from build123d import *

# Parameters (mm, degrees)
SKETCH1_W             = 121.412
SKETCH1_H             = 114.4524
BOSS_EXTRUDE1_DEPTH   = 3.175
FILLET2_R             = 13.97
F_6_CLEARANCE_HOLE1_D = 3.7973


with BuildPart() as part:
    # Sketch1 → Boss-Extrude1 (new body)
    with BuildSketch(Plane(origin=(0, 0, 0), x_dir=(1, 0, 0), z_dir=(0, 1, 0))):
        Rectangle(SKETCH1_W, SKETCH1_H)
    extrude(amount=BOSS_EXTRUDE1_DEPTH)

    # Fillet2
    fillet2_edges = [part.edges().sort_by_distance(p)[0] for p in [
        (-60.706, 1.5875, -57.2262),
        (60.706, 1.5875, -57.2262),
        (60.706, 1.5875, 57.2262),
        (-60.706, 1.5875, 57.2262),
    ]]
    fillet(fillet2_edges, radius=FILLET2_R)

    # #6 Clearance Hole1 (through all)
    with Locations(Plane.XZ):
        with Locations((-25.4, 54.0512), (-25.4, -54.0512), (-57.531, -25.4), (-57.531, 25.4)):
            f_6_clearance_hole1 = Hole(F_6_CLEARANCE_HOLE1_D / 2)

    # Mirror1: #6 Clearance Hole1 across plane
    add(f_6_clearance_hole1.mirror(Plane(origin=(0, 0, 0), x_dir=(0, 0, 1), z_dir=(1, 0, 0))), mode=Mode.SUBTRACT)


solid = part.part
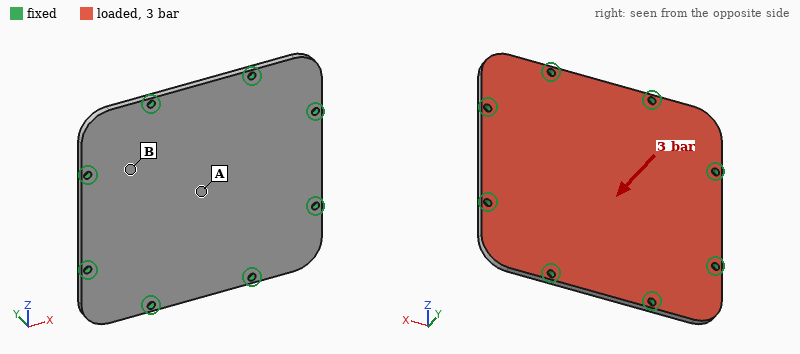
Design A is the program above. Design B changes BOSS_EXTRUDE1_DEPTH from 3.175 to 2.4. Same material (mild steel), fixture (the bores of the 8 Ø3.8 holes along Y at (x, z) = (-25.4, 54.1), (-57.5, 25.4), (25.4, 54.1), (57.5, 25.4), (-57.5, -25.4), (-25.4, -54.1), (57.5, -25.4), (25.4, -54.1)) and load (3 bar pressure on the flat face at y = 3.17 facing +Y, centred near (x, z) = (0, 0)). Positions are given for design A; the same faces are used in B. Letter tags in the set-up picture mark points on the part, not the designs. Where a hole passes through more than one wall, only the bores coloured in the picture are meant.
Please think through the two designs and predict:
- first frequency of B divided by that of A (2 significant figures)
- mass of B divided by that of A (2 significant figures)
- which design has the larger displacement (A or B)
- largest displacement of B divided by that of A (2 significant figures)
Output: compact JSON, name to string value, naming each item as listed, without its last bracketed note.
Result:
{"first frequency of B divided by that of A": "0.77", "mass of B divided by that of A": "0.76", "which design has the larger displacement": "B", "largest displacement of B divided by that of A": "2.2"}
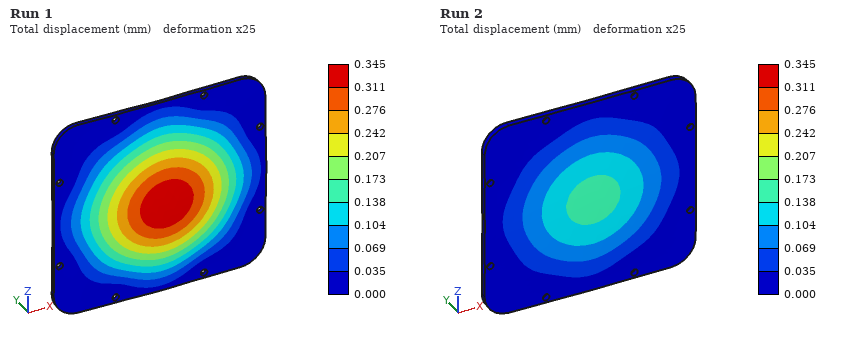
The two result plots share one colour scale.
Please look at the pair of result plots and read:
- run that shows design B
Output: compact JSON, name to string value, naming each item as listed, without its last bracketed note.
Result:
{"run that shows design B": "Run 1"}
